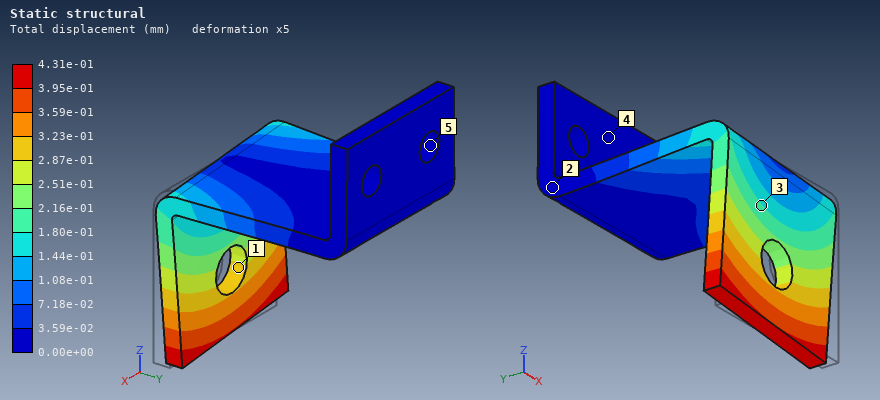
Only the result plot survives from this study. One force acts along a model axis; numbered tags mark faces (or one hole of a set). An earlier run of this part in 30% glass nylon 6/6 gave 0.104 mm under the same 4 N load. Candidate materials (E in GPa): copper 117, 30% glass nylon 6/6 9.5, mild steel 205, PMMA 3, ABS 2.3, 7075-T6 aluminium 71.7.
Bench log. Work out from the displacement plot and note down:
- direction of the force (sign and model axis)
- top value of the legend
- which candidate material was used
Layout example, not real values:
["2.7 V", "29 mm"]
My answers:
["-X", "4.31e-01 mm", "ABS"]
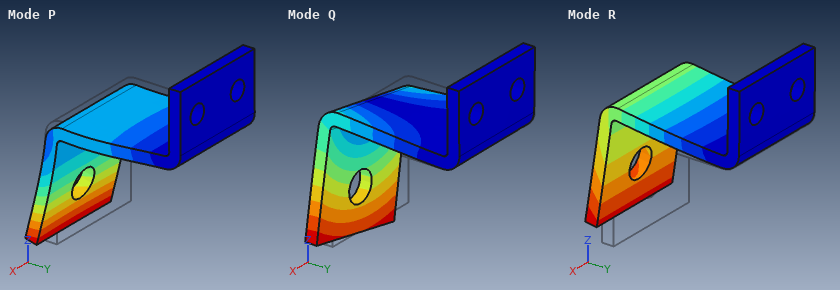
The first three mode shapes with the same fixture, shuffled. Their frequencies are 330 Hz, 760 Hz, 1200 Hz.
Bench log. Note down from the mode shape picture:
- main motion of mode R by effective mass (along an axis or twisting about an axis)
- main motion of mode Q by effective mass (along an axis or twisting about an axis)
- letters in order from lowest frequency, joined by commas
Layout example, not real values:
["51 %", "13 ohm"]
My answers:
["along Z", "along X", "R, Q, P"]
